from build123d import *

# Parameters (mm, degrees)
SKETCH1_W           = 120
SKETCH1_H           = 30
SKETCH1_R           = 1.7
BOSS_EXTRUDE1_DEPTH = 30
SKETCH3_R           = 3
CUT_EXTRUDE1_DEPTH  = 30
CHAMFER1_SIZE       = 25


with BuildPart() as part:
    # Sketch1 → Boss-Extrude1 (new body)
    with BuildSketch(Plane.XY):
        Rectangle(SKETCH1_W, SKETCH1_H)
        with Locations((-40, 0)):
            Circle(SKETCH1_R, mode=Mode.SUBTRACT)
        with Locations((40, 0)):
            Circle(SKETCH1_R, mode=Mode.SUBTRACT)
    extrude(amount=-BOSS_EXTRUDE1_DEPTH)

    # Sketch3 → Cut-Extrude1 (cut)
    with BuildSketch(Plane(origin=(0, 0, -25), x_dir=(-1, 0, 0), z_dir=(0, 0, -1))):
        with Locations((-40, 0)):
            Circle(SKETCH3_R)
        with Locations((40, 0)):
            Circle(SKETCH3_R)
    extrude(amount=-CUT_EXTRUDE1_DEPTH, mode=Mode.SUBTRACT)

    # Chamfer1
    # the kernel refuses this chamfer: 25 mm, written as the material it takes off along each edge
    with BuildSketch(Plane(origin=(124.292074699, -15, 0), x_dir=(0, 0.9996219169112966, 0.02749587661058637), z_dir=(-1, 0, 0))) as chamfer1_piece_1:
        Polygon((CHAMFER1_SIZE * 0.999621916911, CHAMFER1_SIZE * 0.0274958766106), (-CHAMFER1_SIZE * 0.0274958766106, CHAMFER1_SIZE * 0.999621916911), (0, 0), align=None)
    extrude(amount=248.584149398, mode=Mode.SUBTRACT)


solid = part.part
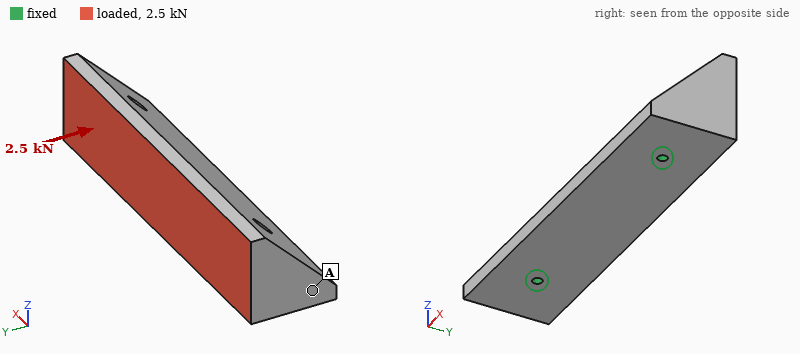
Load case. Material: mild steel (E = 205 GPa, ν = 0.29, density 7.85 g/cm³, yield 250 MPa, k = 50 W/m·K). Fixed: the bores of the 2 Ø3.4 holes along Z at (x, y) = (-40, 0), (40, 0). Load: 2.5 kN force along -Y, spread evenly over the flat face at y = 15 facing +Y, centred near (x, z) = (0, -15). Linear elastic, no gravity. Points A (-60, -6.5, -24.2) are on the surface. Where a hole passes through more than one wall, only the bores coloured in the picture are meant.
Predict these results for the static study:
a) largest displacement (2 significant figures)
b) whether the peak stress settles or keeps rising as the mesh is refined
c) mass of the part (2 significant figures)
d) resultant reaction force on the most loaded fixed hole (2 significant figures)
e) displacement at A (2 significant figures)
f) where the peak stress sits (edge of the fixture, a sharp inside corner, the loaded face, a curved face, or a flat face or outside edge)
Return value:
33 µm
keeps rising
550 g
1.3 kN
7.4 µm
edge of the fixture
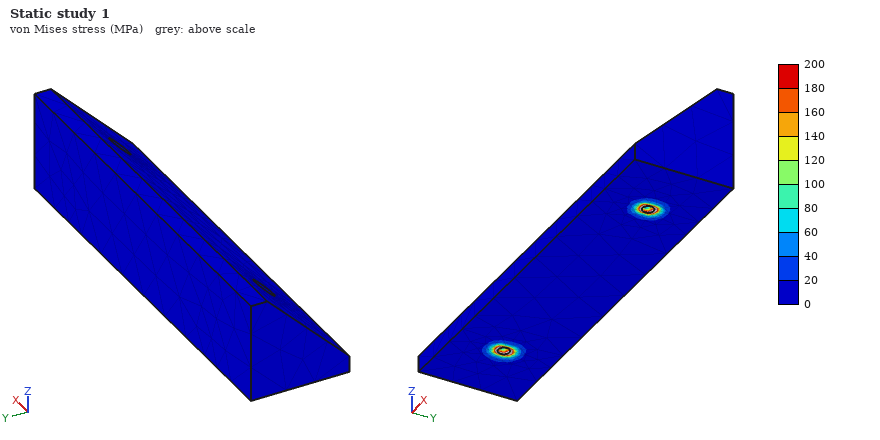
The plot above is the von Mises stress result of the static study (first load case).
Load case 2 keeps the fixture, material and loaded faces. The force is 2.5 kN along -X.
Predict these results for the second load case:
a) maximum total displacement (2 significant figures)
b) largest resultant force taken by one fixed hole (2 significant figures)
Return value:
2.6 µm
1.4 kN
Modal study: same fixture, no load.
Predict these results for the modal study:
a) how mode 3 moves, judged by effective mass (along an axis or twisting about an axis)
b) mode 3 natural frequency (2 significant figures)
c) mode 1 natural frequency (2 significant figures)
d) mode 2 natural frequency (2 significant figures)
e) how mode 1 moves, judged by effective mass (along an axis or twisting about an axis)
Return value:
twisting about Z
7300 Hz
2600 Hz
6800 Hz
along Y
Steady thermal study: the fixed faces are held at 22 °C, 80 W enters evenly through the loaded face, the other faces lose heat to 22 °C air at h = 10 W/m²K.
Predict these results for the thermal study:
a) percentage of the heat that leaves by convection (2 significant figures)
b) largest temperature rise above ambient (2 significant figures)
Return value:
5.5 %
58 K
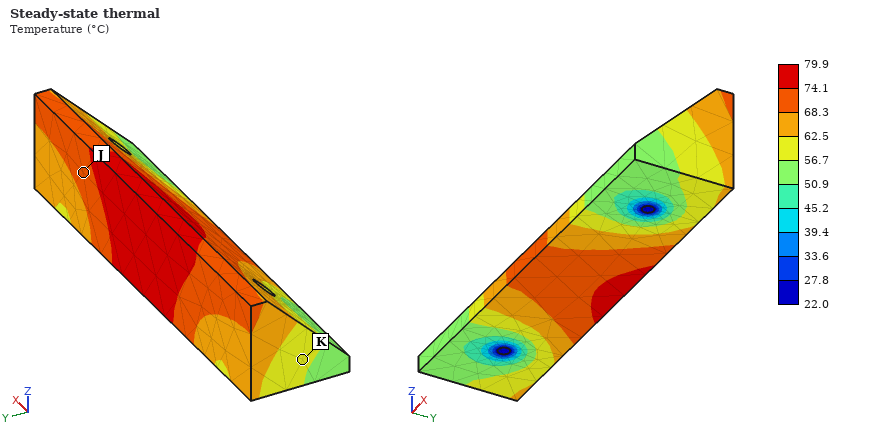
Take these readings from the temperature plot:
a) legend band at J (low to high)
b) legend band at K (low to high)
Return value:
68.3 to 74.1 °C
56.7 to 62.5 °C
